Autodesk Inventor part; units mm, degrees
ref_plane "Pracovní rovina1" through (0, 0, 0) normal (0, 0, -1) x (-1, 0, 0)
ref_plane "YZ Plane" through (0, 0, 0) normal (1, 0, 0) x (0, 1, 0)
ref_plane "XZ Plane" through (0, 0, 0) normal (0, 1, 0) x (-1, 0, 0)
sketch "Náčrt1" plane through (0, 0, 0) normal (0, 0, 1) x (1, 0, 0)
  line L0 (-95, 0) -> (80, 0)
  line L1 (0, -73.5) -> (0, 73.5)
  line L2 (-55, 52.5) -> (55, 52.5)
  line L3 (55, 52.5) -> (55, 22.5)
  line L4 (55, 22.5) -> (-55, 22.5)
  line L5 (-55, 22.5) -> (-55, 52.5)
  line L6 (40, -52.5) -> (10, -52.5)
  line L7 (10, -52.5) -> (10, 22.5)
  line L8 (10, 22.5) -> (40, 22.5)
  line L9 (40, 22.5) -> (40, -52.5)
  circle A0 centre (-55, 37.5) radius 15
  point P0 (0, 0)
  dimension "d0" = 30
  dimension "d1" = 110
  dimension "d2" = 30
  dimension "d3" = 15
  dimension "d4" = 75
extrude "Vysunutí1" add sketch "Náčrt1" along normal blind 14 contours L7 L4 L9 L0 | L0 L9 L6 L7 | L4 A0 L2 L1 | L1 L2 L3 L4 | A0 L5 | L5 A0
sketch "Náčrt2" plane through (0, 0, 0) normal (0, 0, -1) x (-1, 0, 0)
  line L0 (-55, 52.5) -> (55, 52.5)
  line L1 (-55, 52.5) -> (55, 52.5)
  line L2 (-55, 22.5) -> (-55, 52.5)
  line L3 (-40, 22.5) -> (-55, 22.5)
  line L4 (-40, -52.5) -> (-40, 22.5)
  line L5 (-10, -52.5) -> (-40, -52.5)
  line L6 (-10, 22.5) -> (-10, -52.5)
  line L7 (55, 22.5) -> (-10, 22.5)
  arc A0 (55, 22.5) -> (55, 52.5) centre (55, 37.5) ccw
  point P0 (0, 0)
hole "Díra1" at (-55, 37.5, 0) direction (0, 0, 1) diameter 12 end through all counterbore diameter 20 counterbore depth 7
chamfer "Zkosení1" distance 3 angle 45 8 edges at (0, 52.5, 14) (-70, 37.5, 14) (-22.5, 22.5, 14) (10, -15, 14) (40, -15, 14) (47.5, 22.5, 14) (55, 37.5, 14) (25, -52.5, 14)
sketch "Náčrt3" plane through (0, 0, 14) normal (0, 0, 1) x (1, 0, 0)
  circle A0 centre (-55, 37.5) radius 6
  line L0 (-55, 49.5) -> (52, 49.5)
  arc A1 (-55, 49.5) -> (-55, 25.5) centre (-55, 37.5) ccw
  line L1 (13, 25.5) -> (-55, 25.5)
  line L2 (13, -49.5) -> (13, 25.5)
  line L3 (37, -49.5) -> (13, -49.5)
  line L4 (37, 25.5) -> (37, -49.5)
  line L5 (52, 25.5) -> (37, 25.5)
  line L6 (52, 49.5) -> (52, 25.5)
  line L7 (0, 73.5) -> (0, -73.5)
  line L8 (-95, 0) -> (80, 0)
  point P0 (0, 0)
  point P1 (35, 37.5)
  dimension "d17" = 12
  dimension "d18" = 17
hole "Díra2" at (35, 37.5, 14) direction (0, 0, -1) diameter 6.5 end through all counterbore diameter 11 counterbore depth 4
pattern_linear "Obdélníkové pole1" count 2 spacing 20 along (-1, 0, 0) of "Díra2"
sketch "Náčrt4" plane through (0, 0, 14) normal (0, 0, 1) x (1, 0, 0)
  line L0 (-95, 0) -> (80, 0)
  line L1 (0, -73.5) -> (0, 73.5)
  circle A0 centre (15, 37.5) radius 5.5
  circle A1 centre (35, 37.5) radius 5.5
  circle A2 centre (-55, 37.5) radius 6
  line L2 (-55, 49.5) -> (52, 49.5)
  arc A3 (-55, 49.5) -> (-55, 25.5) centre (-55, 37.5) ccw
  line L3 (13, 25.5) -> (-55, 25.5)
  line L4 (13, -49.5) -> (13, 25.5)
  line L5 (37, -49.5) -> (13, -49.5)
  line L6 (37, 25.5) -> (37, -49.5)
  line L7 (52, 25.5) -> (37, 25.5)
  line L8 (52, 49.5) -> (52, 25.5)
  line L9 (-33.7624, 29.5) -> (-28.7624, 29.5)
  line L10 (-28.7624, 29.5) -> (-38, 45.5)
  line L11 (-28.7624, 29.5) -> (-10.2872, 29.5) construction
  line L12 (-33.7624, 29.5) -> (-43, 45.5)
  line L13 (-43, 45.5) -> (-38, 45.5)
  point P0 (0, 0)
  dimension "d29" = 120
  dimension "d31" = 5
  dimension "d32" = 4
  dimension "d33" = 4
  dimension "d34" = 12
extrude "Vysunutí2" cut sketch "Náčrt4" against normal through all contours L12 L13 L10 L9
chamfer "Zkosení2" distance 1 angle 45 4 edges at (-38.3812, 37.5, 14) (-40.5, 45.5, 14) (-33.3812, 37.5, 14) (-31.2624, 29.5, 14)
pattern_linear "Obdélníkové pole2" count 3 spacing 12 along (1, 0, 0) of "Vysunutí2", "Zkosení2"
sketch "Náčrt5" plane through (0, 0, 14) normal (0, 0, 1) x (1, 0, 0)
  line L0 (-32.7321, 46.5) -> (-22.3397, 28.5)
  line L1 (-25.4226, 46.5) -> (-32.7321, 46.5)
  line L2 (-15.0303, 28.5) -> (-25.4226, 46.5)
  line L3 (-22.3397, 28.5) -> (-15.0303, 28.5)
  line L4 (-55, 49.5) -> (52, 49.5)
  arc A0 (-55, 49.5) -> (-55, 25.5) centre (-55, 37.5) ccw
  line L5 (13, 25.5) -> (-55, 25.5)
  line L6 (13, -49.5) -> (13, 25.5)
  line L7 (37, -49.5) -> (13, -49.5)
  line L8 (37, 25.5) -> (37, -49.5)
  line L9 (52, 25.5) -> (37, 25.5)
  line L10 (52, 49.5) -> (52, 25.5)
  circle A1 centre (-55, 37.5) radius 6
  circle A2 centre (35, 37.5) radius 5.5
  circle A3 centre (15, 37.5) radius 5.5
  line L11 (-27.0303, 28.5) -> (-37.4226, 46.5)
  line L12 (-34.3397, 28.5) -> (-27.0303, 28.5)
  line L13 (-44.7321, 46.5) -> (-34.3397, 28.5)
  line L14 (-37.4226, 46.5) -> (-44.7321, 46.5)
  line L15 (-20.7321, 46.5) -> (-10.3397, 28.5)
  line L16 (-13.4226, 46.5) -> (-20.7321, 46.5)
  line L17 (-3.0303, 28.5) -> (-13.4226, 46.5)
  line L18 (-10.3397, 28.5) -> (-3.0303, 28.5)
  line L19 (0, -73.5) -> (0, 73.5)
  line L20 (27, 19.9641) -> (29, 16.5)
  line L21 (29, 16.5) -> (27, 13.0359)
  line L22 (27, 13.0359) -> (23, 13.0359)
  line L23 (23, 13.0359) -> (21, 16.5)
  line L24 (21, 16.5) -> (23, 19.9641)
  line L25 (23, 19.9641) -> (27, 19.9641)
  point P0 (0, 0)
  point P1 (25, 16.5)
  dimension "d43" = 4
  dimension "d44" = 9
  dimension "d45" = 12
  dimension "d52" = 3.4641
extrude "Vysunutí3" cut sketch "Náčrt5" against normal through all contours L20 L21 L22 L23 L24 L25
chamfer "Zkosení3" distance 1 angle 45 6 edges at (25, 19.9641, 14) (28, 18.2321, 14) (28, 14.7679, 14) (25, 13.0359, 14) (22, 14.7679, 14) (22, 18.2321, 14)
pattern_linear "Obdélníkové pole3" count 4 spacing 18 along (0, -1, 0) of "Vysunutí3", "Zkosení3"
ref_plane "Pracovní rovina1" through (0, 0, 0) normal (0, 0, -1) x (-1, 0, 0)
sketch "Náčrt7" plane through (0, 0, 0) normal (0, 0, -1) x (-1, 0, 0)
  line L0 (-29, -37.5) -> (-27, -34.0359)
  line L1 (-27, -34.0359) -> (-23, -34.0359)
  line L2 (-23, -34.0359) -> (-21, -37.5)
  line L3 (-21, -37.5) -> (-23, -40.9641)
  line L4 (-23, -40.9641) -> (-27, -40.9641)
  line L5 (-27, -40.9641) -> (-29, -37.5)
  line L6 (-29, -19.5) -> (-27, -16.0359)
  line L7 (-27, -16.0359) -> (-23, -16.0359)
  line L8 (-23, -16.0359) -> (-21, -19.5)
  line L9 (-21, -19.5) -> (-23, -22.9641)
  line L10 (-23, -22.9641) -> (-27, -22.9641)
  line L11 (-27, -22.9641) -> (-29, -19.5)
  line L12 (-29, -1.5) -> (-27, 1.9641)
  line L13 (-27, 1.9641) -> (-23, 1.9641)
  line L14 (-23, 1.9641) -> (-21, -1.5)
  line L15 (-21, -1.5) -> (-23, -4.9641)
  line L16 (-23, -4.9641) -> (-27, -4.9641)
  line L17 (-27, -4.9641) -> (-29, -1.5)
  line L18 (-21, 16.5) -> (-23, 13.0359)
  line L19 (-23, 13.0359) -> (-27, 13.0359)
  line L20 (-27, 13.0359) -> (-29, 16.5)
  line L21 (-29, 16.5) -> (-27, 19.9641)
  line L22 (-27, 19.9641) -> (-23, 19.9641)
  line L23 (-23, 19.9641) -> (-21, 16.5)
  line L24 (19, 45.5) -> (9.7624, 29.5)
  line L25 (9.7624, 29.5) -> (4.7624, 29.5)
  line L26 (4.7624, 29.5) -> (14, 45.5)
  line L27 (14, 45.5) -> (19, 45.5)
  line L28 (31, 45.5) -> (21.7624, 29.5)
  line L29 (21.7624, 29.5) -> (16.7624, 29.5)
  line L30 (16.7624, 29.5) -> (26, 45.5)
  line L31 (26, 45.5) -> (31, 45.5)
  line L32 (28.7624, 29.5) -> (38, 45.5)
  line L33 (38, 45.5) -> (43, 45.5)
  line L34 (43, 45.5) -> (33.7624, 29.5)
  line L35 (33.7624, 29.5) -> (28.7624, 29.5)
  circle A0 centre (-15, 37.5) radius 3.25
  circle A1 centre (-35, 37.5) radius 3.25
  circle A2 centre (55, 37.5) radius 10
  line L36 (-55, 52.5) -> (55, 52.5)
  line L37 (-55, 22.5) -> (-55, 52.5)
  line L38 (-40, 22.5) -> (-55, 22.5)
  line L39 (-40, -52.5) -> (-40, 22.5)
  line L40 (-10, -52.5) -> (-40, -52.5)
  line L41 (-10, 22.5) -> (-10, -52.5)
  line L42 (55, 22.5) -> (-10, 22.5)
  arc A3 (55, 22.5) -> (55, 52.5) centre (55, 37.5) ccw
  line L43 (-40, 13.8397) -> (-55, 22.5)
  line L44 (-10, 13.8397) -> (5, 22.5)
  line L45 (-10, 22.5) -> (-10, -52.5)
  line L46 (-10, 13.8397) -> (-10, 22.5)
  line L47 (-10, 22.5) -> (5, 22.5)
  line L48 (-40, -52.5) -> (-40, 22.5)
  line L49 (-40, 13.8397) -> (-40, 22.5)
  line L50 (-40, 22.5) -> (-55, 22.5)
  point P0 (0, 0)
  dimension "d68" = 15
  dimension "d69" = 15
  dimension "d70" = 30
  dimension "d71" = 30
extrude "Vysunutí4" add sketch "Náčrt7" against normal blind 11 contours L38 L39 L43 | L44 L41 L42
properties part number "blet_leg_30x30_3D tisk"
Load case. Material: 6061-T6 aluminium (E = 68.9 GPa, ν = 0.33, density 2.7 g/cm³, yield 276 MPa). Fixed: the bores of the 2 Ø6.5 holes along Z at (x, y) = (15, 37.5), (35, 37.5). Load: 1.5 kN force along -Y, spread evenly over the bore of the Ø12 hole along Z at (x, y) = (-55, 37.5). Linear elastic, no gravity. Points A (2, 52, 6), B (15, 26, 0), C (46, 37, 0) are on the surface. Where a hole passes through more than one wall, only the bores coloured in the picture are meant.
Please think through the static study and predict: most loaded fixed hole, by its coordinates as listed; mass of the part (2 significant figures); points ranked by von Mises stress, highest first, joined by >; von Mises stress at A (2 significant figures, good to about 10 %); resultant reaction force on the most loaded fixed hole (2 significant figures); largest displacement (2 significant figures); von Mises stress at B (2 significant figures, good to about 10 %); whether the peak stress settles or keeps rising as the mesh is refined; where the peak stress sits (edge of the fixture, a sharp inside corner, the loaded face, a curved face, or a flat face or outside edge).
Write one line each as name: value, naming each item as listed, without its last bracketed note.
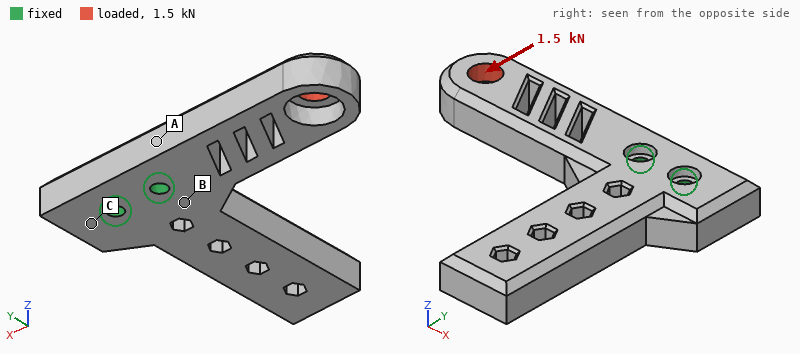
most loaded fixed hole, by its coordinates as listed: (15, 37.5)
mass of the part: 190 g
points ranked by von Mises stress, highest first, joined by >: A > B > C
von Mises stress at A: 40 MPa
resultant reaction force on the most loaded fixed hole: 5.2 kN
largest displacement: 0.20 mm
von Mises stress at B: 29 MPa
whether the peak stress settles or keeps rising as the mesh is refined: keeps rising
where the peak stress sits: edge of the fixture
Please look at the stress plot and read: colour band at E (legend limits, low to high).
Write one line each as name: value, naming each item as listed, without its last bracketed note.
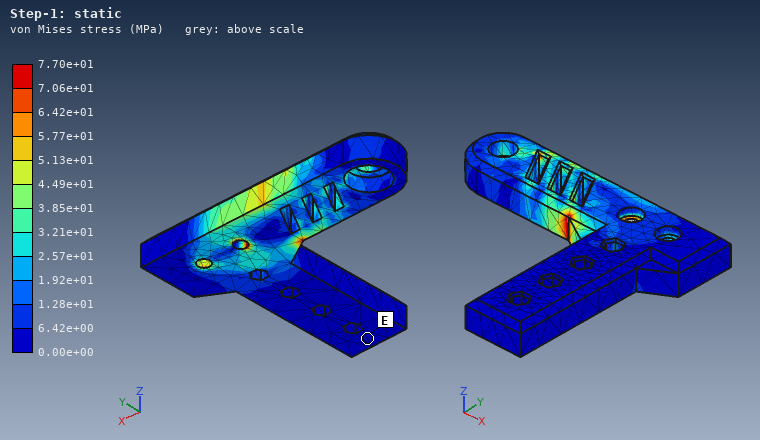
colour band at E: 0.00e+00 to 6.42e+00 MPa
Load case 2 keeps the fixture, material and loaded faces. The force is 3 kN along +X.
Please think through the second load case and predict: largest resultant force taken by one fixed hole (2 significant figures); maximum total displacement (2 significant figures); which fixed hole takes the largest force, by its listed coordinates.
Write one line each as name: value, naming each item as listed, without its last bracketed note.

largest resultant force taken by one fixed hole: 2.1 kN
maximum total displacement: 0.16 mm
which fixed hole takes the largest force, by its listed coordinates: (15, 37.5)
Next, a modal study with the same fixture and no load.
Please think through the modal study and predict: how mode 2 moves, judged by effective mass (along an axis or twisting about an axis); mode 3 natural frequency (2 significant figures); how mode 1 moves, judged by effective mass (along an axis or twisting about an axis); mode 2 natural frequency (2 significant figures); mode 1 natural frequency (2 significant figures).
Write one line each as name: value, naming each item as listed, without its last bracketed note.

how mode 2 moves, judged by effective mass: along Z
mode 3 natural frequency: 2700 Hz
how mode 1 moves, judged by effective mass: along Z
mode 2 natural frequency: 1600 Hz
mode 1 natural frequency: 1400 Hz
